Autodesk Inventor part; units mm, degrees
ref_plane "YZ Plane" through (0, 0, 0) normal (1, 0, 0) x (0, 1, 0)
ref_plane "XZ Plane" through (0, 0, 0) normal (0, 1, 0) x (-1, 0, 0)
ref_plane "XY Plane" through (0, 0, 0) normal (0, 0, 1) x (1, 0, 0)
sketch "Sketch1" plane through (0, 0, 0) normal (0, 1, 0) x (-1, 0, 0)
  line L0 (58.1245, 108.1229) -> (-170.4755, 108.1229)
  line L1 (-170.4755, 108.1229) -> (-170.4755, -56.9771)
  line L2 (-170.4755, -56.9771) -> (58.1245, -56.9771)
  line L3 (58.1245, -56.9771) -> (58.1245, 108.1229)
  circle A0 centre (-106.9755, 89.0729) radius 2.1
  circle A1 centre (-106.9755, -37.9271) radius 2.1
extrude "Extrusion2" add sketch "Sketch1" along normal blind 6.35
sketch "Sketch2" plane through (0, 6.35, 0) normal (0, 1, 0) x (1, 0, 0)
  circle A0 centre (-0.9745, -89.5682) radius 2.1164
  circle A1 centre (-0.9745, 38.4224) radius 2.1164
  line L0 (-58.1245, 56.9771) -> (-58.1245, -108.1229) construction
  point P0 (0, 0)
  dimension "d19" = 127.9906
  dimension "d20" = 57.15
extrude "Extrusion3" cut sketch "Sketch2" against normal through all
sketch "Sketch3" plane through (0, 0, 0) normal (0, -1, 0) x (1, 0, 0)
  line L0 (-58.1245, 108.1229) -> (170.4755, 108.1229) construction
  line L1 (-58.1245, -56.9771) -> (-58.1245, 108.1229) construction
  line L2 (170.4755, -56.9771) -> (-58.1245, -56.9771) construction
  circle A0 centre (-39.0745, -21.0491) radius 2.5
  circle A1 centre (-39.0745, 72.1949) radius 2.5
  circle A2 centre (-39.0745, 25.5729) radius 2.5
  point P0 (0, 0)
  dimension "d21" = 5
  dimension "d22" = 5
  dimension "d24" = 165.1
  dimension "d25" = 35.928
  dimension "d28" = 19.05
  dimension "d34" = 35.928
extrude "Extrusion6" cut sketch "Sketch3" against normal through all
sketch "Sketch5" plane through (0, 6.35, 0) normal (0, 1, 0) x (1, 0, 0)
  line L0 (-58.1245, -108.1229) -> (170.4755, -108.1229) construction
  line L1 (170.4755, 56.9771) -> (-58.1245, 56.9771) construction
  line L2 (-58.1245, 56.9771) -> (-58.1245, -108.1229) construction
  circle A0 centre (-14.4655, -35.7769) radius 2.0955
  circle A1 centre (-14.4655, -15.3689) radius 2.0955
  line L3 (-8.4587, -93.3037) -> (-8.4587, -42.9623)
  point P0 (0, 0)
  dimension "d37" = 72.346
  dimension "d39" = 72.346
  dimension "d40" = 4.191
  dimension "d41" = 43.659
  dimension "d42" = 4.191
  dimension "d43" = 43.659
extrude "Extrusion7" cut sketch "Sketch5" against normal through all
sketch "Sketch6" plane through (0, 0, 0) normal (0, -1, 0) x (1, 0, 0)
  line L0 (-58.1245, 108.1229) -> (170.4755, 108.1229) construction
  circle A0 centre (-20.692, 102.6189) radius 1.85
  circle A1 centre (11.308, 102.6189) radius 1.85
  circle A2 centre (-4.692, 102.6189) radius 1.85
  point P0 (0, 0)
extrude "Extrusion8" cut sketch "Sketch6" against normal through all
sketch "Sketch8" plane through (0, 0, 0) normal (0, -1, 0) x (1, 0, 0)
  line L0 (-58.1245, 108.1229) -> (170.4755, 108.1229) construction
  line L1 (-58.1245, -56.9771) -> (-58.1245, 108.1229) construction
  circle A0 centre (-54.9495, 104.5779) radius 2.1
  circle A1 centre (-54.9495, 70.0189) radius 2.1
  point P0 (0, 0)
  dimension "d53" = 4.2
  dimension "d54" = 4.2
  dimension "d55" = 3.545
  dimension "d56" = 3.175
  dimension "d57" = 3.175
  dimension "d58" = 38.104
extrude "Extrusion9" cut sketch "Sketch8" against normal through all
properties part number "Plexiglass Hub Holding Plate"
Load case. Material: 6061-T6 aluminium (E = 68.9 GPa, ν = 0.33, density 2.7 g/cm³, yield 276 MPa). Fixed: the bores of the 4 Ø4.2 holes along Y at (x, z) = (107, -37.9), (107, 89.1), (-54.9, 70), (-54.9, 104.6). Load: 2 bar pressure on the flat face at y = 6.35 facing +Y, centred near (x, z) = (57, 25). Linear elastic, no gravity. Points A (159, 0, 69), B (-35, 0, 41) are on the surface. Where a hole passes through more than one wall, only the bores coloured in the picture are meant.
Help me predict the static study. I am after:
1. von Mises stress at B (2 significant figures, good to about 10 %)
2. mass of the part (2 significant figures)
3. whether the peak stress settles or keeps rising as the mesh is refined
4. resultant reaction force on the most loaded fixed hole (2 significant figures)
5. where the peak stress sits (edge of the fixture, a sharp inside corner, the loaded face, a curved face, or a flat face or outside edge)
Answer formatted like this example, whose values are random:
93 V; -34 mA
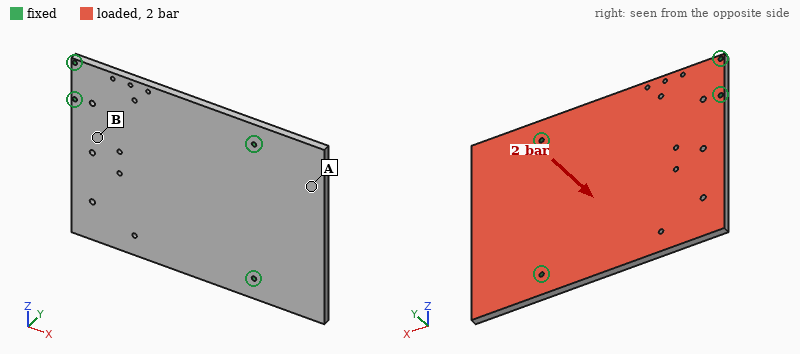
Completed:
76 MPa; 640 g; keeps rising; 3.1 kN; edge of the fixture
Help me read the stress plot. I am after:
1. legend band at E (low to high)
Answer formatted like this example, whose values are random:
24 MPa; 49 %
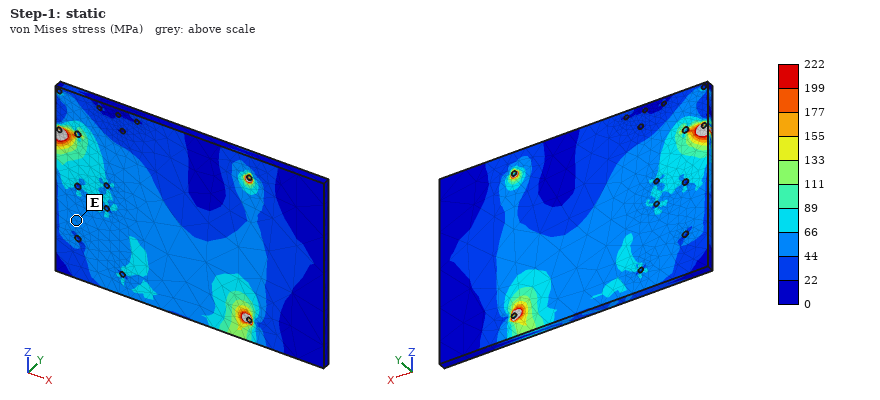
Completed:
44 to 66 MPa
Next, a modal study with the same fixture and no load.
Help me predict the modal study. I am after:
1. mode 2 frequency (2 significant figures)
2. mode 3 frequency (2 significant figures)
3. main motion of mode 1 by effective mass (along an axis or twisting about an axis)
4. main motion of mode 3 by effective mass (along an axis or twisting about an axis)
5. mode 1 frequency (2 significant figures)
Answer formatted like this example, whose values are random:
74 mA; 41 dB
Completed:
870 Hz; 1100 Hz; along Y; along Y; 440 Hz
